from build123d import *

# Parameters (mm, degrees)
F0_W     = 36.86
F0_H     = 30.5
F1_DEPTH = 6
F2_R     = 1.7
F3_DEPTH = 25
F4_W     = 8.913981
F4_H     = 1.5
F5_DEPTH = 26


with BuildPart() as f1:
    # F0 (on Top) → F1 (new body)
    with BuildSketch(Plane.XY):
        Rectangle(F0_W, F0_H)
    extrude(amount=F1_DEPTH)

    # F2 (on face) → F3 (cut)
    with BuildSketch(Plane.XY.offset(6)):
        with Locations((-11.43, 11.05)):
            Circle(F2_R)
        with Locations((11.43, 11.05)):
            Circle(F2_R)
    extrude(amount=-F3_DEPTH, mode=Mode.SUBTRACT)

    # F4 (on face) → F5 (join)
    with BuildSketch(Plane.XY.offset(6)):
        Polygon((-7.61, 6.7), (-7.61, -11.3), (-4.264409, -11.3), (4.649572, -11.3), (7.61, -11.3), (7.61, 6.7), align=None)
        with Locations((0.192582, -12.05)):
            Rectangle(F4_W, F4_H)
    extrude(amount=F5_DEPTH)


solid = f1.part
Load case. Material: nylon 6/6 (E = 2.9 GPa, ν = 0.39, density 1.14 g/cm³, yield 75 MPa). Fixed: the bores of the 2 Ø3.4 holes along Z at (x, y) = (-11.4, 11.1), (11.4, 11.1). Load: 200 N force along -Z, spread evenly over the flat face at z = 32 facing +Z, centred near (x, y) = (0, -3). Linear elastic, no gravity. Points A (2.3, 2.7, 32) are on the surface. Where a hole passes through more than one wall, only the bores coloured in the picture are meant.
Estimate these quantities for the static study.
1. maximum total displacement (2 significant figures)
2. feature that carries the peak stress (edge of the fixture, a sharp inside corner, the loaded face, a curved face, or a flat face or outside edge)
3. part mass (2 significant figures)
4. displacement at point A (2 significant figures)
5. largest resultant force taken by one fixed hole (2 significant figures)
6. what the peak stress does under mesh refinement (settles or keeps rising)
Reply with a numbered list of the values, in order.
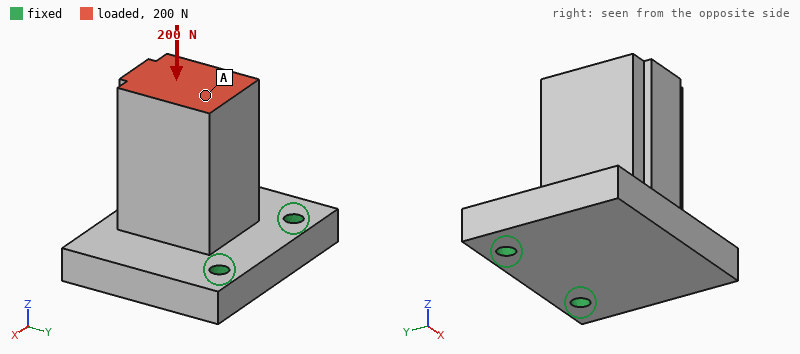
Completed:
1. 0.42 mm
2. edge of the fixture
3. 16 g
4. 0.34 mm
5. 100 N
6. keeps rising
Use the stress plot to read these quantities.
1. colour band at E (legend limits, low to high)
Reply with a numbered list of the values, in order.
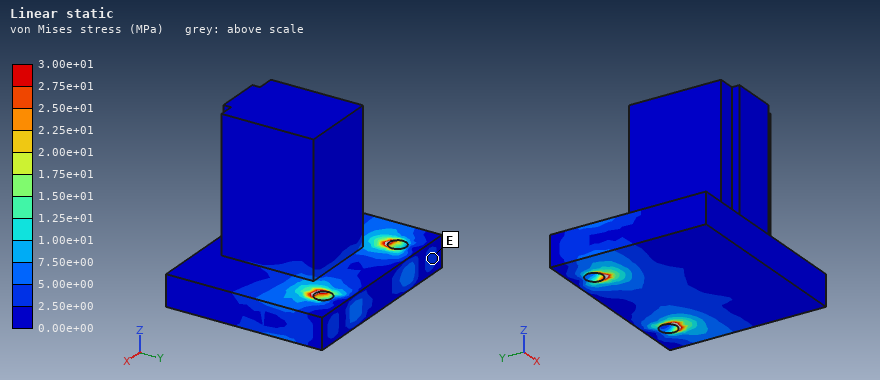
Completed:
1. 2.50e+00 to 5.00e+00 MPa
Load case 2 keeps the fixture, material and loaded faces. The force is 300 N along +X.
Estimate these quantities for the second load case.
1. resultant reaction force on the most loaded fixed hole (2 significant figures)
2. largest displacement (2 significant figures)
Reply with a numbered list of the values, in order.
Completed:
1. 450 N
2. 0.53 mm
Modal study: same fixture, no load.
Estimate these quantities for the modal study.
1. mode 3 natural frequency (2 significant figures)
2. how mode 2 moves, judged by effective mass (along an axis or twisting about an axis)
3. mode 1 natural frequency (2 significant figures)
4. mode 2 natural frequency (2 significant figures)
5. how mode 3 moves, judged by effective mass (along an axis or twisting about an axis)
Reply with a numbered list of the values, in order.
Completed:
1. 4300 Hz
2. along X
3. 960 Hz
4. 2100 Hz
5. along Z
